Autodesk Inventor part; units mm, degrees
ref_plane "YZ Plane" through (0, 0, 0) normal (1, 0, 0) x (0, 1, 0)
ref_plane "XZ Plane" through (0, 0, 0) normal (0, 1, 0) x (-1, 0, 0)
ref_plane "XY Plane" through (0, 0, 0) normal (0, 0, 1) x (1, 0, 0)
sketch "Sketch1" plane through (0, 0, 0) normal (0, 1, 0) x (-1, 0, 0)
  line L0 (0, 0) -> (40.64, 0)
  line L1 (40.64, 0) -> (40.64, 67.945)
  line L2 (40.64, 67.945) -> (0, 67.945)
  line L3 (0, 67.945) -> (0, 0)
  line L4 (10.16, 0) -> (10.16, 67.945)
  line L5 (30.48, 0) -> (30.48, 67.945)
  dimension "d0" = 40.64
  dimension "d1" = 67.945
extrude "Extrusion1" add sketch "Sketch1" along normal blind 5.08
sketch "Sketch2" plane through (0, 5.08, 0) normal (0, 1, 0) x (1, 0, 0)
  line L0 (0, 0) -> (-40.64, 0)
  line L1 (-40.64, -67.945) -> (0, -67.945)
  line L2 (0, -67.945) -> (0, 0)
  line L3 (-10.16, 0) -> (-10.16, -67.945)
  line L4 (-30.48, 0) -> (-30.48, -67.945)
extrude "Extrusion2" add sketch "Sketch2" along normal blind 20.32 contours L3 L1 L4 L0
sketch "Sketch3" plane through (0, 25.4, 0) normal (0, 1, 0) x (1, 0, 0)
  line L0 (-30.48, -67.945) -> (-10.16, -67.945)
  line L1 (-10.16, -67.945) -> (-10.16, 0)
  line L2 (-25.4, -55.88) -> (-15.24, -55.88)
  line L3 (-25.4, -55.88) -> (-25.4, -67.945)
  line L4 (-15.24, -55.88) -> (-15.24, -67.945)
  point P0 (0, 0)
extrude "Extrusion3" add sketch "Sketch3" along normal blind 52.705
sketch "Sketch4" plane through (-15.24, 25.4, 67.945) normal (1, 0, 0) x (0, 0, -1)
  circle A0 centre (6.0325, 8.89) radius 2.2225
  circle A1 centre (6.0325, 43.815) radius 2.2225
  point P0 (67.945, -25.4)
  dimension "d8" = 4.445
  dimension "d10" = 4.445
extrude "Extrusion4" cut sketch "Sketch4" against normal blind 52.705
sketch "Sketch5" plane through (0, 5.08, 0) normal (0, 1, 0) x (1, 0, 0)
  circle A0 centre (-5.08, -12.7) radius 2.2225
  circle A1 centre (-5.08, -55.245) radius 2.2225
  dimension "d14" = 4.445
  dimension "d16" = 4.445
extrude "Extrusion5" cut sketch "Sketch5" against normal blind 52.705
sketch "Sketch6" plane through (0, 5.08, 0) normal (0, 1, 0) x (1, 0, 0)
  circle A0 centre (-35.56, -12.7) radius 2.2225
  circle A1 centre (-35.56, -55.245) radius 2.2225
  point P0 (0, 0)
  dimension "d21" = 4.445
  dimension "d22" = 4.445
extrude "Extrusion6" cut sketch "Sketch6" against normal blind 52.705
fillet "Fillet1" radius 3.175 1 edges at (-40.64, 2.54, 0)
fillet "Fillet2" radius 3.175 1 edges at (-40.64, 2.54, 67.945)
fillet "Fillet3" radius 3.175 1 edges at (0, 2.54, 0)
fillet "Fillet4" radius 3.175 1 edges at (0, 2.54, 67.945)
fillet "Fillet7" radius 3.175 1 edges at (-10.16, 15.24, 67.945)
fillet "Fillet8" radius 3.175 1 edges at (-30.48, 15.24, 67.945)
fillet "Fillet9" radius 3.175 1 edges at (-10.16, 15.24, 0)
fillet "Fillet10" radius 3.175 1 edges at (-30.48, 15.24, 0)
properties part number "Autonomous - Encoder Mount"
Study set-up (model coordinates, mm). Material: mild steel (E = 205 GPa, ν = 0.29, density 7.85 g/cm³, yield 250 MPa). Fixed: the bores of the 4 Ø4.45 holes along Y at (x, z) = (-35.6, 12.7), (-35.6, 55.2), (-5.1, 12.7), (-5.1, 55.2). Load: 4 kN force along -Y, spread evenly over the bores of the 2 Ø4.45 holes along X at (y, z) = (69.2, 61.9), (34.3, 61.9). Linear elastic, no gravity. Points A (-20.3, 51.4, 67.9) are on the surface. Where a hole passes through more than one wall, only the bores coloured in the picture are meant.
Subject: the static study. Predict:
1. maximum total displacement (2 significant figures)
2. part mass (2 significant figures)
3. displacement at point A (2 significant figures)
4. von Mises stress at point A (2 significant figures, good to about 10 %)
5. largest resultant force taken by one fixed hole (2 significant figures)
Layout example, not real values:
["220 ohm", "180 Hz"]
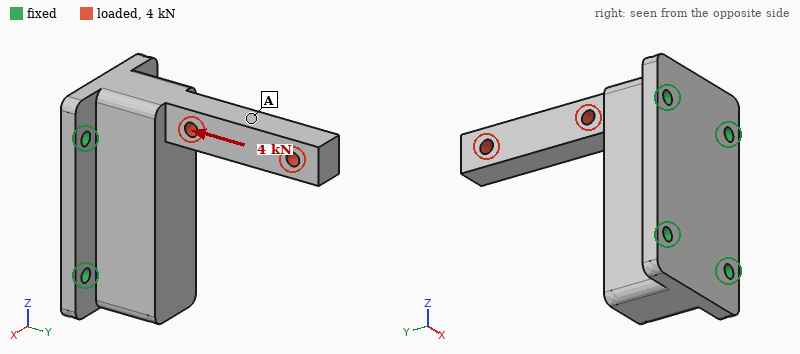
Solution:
["23 µm", "370 g", "17 µm", "16 MPa", "2.4 kN"]
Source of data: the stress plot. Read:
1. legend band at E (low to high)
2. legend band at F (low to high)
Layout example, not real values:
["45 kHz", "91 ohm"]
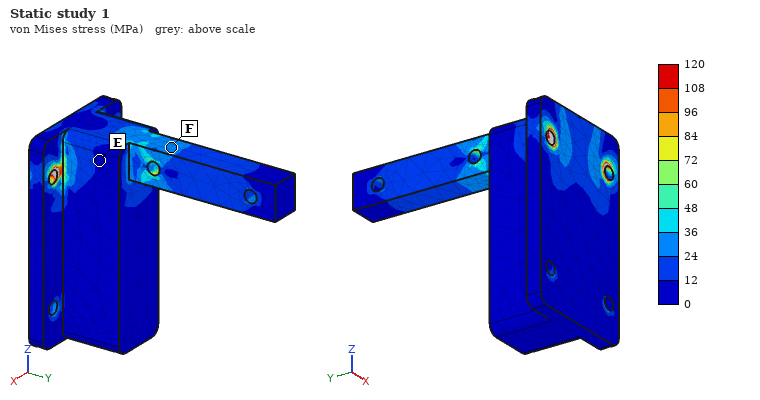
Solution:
["0 to 12 MPa", "24 to 36 MPa"]
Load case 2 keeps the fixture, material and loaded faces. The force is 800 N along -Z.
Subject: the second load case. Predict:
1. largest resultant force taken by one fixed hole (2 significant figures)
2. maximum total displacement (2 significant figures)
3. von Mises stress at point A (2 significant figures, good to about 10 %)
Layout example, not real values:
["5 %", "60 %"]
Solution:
["600 N", "83 µm", "29 MPa"]
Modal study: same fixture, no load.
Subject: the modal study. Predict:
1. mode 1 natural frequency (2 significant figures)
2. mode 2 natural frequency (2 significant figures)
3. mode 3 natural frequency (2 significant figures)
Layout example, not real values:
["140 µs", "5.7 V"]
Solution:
["2300 Hz", "2800 Hz", "9500 Hz"]
